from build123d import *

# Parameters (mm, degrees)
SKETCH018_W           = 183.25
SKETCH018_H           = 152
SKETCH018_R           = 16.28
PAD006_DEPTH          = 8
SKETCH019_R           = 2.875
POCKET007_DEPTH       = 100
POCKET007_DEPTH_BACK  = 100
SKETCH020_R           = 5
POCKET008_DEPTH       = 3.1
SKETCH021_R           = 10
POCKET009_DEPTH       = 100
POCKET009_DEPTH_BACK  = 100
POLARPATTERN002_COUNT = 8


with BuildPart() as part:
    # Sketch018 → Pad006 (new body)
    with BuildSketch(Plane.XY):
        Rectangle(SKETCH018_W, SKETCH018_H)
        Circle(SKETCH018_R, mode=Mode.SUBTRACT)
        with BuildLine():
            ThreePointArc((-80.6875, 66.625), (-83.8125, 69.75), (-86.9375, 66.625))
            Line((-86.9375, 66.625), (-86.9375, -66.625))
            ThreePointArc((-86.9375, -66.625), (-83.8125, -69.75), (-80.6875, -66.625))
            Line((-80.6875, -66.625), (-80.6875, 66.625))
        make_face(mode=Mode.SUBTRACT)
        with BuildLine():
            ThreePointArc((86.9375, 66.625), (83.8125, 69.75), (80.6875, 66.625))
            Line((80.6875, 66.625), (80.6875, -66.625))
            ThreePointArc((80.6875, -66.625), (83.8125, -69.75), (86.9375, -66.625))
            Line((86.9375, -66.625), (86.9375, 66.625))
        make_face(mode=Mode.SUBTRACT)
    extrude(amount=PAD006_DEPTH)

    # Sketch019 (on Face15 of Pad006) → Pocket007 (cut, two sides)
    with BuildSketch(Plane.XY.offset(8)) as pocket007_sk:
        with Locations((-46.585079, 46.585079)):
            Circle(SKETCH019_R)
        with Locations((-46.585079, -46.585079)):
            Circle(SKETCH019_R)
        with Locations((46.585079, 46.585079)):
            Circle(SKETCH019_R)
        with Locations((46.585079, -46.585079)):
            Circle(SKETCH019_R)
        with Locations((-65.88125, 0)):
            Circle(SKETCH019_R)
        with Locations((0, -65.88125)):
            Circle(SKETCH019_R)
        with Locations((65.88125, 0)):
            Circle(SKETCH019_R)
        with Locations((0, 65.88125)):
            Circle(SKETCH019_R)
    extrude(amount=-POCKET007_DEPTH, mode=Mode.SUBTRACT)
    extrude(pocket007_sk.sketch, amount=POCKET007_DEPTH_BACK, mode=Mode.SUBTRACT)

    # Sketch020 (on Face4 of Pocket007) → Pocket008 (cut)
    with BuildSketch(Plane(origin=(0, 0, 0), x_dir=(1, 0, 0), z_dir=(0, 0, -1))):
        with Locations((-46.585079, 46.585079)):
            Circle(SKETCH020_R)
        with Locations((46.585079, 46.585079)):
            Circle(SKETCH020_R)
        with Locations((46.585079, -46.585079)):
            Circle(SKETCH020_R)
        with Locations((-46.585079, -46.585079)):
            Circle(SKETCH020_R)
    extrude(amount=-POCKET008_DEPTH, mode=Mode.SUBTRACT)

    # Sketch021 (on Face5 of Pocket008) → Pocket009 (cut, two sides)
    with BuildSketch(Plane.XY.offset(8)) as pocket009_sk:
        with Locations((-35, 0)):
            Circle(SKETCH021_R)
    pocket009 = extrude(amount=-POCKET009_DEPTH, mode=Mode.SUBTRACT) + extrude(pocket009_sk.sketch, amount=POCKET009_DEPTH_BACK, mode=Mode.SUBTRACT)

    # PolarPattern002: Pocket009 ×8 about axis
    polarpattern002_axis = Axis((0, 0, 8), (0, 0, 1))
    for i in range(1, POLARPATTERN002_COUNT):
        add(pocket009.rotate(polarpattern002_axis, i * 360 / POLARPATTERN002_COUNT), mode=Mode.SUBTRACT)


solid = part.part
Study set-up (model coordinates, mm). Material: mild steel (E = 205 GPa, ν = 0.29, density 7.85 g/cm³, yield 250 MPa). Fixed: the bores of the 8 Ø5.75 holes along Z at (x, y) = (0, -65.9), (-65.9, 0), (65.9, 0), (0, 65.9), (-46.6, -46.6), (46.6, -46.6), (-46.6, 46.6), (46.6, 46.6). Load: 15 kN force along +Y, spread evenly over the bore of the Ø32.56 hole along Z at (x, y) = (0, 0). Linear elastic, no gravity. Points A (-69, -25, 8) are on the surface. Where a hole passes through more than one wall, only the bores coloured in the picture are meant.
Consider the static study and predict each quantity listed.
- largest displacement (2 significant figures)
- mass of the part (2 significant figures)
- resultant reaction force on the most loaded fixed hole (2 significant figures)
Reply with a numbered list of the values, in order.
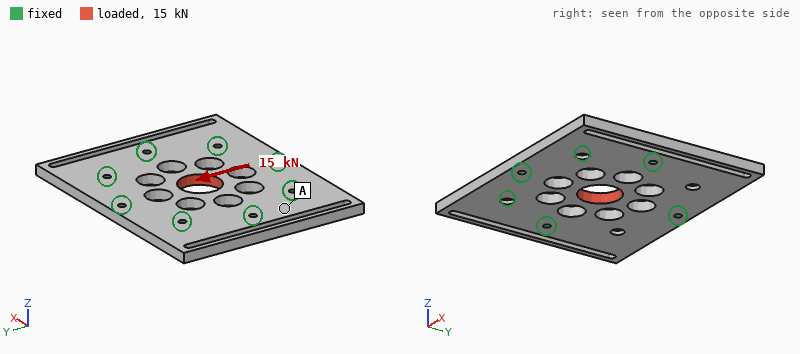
1. 8.3 µm
2. 1.4 kg
3. 3.1 kN
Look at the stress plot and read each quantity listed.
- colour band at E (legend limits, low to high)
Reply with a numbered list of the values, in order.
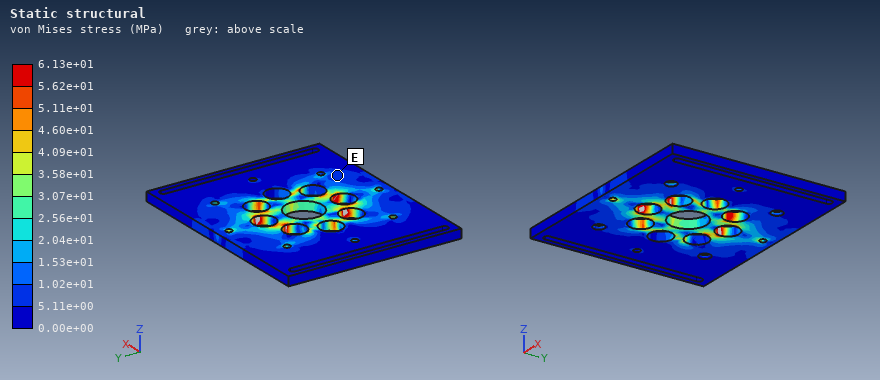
1. 5.11e+00 to 1.02e+01 MPa
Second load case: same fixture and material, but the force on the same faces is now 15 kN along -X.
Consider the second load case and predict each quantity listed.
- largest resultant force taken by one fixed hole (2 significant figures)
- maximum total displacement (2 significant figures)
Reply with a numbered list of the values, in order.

1. 3.2 kN
2. 8.2 µm
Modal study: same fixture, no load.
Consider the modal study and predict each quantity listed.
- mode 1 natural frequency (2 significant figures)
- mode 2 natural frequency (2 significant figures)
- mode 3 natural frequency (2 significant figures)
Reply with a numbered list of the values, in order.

1. 1200 Hz
2. 1200 Hz
3. 1500 Hz
